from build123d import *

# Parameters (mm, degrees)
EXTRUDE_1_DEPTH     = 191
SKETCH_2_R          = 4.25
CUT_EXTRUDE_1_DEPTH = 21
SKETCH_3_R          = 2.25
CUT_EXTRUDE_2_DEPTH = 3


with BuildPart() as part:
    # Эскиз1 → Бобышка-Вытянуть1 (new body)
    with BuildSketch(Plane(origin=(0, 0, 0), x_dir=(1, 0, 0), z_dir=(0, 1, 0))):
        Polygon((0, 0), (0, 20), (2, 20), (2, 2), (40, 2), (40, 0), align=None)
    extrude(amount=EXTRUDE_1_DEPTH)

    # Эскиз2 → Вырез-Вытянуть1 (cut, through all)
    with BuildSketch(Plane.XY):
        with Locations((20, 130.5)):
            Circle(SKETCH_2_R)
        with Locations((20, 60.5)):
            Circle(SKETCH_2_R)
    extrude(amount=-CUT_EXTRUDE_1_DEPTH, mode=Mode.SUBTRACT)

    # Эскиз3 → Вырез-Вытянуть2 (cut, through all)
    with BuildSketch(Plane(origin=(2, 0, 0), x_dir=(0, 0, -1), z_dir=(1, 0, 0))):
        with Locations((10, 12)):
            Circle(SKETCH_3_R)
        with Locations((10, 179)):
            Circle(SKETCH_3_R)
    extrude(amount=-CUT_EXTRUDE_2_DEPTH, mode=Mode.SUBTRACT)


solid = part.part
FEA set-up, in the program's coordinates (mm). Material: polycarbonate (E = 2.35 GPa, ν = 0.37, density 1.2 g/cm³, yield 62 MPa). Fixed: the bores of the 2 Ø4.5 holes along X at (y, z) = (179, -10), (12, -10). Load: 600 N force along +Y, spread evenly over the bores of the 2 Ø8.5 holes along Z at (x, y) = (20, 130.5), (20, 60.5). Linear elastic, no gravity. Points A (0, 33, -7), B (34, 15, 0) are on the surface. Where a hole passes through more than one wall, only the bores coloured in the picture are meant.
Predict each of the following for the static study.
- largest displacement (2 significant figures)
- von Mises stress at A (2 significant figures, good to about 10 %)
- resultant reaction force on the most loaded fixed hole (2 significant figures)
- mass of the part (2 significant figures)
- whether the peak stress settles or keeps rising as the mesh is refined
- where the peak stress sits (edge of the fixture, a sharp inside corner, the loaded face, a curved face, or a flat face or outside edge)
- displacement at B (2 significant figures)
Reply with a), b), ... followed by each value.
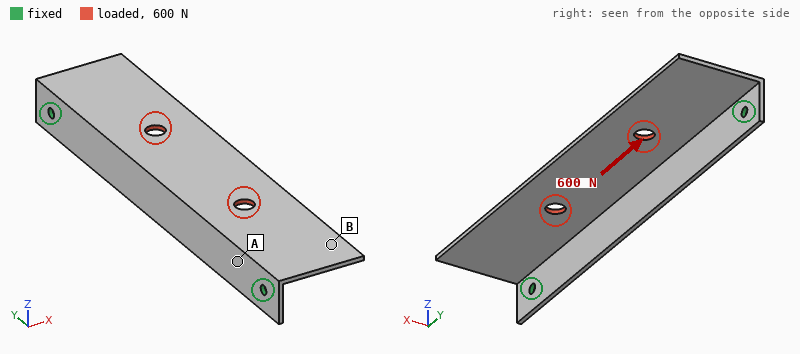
a) 1.6 mm
b) 4.5 MPa
c) 310 N
d) 26 g
e) keeps rising
f) edge of the fixture
g) 1.2 mm
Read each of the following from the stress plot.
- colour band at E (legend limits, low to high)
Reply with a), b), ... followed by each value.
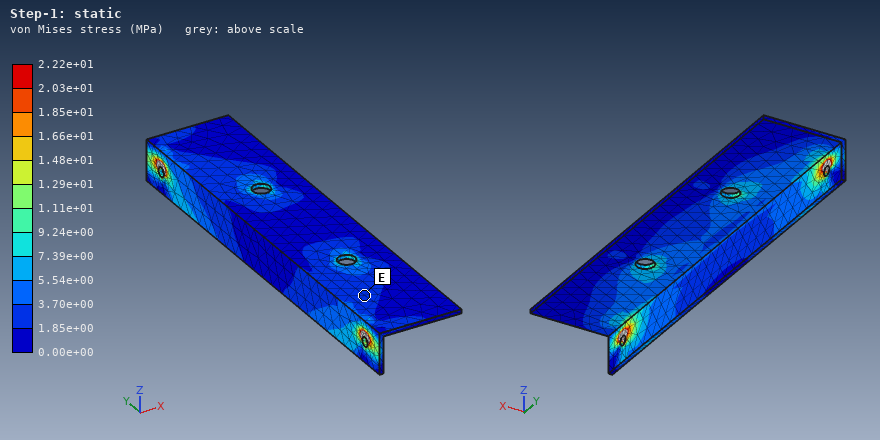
a) 1.85e+00 to 3.70e+00 MPa
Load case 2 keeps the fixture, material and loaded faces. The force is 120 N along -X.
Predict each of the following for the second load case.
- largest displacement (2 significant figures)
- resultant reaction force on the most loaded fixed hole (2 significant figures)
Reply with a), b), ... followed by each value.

a) 1.9 mm
b) 81 N
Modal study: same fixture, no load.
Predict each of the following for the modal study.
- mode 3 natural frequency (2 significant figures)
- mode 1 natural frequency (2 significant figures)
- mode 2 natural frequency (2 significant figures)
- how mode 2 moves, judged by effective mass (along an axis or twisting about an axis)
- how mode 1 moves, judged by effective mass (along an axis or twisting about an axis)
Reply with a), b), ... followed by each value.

a) 310 Hz
b) 120 Hz
c) 230 Hz
d) twisting about X
e) along Z
